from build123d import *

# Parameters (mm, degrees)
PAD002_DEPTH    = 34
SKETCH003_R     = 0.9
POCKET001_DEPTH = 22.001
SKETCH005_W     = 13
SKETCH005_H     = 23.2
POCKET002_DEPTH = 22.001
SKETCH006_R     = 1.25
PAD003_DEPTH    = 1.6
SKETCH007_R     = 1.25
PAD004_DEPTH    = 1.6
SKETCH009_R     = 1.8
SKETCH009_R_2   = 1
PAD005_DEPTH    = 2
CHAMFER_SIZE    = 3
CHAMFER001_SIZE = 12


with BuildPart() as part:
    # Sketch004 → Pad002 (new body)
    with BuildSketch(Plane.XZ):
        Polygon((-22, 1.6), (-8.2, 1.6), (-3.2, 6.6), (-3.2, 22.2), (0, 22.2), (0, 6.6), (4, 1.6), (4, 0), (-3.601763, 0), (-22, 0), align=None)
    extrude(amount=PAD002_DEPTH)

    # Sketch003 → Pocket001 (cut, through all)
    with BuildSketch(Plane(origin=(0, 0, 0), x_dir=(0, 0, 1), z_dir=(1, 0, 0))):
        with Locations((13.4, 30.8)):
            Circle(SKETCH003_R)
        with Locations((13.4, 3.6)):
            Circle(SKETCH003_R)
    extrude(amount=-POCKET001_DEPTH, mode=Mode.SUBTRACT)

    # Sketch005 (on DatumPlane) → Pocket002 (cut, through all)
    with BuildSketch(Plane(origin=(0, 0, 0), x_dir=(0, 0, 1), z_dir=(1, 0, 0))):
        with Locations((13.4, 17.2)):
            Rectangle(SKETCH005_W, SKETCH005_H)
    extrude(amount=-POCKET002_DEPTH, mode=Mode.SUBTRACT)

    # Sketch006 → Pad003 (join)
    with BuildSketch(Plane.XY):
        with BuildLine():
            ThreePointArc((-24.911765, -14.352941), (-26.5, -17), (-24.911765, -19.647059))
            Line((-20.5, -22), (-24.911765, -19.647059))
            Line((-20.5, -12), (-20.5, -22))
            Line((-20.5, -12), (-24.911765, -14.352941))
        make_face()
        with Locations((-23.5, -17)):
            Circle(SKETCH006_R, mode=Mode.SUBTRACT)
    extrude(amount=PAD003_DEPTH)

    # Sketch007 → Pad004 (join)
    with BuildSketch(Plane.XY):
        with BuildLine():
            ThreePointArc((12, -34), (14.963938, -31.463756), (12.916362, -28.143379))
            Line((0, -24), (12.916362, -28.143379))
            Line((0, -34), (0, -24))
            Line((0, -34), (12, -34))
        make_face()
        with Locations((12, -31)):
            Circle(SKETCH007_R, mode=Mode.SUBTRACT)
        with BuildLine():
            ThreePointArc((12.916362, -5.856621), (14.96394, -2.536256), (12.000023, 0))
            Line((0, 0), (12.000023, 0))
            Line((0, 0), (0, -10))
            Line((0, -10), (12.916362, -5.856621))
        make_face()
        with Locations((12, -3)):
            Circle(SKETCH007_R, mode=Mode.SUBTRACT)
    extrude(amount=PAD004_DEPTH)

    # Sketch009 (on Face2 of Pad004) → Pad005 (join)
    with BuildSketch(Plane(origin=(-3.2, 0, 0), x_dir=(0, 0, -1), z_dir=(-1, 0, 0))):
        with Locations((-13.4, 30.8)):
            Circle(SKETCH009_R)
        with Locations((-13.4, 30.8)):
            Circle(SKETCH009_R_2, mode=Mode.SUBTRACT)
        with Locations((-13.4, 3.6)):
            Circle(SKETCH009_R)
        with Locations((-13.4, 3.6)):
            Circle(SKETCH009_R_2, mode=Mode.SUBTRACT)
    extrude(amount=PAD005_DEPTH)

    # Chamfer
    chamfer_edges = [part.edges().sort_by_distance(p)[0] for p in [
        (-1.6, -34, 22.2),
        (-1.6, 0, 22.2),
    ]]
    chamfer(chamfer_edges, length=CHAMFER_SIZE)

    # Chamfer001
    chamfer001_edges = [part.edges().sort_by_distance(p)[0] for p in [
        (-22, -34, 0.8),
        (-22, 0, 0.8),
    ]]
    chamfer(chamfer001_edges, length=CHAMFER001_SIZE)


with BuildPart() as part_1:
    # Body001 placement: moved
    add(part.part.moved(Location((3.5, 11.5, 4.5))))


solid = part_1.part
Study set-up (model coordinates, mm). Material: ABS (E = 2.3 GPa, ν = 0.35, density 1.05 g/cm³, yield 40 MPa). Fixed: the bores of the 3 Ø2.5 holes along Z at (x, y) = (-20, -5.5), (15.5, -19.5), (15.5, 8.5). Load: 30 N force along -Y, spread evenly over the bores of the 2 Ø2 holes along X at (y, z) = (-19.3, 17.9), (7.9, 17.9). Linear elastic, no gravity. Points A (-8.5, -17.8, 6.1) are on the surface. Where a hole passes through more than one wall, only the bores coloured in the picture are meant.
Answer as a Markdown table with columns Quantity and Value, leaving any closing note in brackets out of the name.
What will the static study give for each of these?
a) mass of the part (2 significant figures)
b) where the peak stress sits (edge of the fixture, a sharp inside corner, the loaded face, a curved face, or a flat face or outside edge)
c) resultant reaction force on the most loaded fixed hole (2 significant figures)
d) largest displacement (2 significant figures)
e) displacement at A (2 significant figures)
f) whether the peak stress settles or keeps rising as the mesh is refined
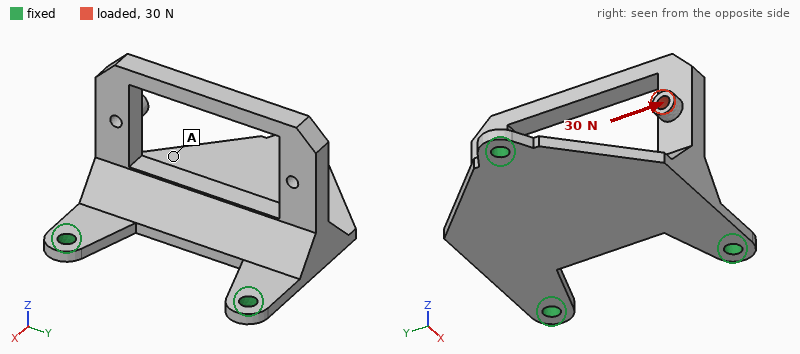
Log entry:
| Quantity | Value |
|---|---|
| mass of the part | 3.6 g |
| where the peak stress sits | edge of the fixture |
| resultant reaction force on the most loaded fixed hole | 18 N |
| largest displacement | 0.36 mm |
| displacement at A | 0.13 mm |
| whether the peak stress settles or keeps rising as the mesh is refined | keeps rising |
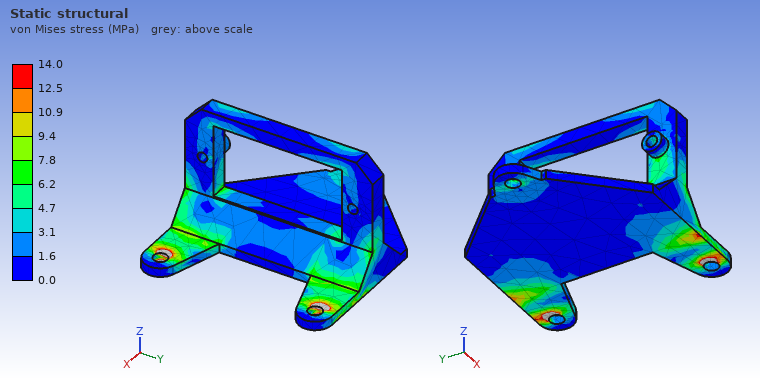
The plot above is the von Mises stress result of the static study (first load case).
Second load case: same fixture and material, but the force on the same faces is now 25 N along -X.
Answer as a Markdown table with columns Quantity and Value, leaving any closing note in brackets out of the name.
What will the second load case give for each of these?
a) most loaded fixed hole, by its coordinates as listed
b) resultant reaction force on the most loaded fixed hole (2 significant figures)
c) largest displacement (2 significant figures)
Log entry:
| Quantity | Value |
|---|---|
| most loaded fixed hole, by its coordinates as listed | (-20, -5.5) |
| resultant reaction force on the most loaded fixed hole | 16 N |
| largest displacement | 0.53 mm |
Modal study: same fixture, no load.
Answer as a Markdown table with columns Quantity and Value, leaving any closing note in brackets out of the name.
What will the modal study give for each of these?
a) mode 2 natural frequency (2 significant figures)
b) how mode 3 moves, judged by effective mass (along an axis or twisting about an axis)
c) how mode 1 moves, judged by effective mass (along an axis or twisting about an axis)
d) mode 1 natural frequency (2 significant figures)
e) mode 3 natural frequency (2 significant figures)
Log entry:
| Quantity | Value |
|---|---|
| mode 2 natural frequency | 1200 Hz |
| how mode 3 moves, judged by effective mass | along Z |
| how mode 1 moves, judged by effective mass | along Z |
| mode 1 natural frequency | 980 Hz |
| mode 3 natural frequency | 1600 Hz |
